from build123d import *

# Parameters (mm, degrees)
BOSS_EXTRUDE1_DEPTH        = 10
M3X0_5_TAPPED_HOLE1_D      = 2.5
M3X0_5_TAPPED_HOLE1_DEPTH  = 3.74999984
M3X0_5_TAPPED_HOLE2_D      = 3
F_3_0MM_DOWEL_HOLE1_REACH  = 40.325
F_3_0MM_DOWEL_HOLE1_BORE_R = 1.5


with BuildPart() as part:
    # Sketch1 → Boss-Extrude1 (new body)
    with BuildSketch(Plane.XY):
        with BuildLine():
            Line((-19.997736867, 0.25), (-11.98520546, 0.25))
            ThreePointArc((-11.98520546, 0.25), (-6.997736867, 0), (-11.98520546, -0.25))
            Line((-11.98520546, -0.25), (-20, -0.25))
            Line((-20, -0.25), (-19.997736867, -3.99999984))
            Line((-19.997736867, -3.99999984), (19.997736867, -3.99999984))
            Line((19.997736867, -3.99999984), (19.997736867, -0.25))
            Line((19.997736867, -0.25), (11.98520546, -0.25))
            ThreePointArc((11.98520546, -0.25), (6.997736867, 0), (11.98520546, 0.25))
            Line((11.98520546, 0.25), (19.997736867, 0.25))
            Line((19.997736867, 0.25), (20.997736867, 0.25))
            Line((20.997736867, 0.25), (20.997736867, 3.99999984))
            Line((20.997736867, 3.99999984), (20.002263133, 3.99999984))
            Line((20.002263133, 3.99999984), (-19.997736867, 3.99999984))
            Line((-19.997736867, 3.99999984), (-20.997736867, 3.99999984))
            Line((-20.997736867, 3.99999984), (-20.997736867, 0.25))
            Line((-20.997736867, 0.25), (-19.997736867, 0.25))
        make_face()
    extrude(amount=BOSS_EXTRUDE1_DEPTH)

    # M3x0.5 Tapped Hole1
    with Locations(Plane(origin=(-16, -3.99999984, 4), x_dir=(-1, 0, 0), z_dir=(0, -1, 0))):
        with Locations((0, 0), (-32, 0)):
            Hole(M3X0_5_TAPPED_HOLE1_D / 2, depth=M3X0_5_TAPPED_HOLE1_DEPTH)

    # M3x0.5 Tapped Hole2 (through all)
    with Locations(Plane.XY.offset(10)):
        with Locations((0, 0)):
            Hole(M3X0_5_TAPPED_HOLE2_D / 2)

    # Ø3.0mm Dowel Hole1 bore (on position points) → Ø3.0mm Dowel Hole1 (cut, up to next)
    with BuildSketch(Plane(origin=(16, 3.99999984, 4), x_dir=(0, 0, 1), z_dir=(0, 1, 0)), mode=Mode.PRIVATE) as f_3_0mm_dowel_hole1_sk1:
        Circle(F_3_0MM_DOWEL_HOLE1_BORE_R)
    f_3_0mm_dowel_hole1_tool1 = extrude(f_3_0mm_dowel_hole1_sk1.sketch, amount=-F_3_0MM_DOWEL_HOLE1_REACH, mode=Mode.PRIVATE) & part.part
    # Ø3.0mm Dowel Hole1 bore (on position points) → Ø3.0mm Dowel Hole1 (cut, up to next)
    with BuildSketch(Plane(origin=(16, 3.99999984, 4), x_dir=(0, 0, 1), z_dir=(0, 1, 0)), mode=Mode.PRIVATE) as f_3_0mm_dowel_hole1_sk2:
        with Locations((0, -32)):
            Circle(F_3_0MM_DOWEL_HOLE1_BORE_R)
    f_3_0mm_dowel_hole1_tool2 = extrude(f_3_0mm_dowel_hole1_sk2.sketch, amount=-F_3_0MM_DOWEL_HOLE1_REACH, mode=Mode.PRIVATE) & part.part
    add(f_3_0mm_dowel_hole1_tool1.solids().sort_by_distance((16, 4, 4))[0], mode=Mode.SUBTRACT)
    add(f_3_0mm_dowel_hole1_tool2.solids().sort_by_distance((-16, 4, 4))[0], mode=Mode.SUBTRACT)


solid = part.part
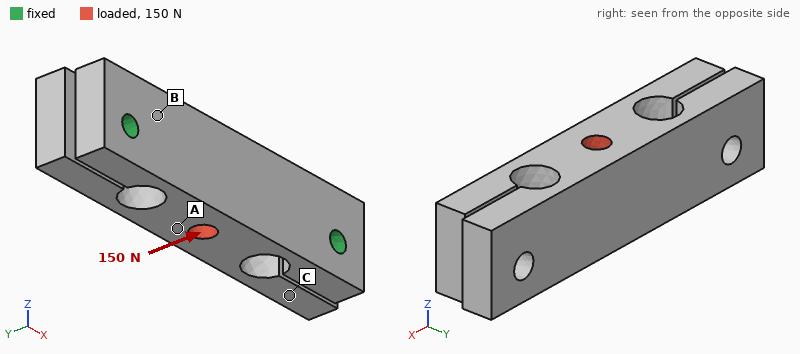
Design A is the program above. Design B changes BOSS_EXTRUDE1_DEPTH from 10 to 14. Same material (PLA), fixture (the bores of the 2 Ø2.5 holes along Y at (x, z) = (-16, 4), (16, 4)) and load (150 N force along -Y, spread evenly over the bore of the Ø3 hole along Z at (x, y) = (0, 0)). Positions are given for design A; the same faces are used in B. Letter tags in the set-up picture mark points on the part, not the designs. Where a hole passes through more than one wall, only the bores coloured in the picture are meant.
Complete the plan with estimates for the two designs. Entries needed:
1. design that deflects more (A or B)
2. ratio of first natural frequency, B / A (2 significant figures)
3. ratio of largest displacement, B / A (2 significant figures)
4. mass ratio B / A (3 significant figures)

B
0.98
1.2
1.41
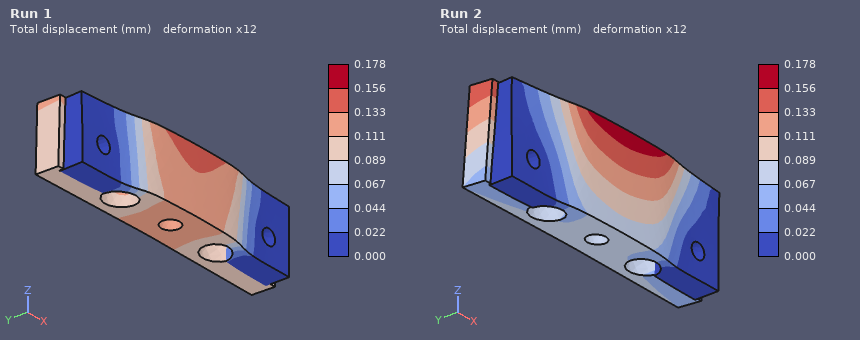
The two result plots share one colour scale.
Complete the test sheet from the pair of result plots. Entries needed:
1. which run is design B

Run 2
